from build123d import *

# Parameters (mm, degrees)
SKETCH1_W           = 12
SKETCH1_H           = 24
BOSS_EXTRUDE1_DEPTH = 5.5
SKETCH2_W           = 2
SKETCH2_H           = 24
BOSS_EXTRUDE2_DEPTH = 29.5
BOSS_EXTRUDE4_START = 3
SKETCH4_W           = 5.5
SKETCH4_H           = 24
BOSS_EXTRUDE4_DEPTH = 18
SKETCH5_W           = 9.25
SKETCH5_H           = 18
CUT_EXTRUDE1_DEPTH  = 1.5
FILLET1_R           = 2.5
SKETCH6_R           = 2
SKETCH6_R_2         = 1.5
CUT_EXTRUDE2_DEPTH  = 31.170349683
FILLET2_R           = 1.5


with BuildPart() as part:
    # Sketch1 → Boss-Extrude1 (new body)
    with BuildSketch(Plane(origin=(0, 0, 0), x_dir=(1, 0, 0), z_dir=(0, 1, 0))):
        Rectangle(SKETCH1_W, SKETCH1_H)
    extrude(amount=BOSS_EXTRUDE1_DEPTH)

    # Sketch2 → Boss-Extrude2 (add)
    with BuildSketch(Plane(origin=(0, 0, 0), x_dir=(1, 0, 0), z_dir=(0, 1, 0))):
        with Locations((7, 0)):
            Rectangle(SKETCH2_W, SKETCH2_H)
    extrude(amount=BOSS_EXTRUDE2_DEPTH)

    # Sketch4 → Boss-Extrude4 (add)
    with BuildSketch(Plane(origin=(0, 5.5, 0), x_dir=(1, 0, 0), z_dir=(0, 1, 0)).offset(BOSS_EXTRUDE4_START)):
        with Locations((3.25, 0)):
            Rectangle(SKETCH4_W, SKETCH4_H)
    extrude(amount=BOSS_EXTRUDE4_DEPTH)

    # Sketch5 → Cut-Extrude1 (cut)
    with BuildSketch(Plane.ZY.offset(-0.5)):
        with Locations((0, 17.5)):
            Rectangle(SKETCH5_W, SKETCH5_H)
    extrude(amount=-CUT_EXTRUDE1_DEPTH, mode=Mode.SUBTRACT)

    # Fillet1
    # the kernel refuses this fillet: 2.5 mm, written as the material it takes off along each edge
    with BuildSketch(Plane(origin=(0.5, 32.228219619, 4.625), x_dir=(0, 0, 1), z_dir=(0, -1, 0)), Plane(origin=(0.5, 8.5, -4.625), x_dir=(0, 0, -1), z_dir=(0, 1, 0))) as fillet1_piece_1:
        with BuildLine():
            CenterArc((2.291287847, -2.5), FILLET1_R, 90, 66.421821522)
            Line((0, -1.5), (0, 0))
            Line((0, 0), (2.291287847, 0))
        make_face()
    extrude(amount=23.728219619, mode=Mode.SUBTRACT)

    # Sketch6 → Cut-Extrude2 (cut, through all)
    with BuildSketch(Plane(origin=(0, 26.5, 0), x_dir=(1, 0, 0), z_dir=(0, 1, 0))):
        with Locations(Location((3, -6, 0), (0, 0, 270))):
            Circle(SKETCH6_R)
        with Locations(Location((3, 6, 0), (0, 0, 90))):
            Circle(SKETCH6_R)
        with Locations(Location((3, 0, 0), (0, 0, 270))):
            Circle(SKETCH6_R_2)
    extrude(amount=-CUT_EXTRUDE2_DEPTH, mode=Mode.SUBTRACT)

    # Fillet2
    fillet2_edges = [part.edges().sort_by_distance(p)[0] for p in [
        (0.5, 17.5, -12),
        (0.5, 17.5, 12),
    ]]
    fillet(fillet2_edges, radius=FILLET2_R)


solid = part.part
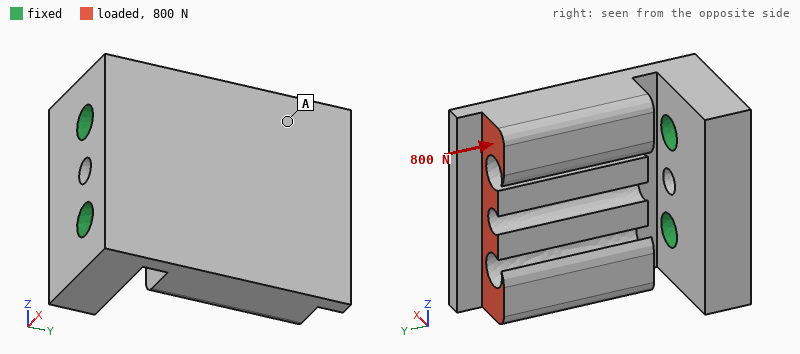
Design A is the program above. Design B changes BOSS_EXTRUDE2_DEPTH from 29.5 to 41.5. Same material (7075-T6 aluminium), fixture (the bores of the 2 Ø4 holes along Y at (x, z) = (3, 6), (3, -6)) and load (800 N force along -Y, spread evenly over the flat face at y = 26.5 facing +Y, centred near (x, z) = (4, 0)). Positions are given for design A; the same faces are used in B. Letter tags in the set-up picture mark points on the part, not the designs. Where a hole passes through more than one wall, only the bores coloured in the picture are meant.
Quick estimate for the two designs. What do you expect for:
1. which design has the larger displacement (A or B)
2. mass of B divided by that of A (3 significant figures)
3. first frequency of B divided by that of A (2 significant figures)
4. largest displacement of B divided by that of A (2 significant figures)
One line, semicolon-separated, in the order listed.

B; 1.13; 0.67; 1.6
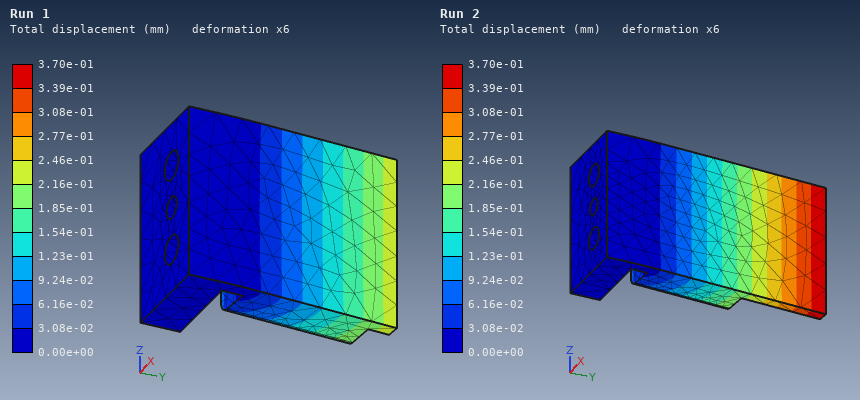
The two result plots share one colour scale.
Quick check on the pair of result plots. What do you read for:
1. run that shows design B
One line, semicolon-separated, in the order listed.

Run 2
